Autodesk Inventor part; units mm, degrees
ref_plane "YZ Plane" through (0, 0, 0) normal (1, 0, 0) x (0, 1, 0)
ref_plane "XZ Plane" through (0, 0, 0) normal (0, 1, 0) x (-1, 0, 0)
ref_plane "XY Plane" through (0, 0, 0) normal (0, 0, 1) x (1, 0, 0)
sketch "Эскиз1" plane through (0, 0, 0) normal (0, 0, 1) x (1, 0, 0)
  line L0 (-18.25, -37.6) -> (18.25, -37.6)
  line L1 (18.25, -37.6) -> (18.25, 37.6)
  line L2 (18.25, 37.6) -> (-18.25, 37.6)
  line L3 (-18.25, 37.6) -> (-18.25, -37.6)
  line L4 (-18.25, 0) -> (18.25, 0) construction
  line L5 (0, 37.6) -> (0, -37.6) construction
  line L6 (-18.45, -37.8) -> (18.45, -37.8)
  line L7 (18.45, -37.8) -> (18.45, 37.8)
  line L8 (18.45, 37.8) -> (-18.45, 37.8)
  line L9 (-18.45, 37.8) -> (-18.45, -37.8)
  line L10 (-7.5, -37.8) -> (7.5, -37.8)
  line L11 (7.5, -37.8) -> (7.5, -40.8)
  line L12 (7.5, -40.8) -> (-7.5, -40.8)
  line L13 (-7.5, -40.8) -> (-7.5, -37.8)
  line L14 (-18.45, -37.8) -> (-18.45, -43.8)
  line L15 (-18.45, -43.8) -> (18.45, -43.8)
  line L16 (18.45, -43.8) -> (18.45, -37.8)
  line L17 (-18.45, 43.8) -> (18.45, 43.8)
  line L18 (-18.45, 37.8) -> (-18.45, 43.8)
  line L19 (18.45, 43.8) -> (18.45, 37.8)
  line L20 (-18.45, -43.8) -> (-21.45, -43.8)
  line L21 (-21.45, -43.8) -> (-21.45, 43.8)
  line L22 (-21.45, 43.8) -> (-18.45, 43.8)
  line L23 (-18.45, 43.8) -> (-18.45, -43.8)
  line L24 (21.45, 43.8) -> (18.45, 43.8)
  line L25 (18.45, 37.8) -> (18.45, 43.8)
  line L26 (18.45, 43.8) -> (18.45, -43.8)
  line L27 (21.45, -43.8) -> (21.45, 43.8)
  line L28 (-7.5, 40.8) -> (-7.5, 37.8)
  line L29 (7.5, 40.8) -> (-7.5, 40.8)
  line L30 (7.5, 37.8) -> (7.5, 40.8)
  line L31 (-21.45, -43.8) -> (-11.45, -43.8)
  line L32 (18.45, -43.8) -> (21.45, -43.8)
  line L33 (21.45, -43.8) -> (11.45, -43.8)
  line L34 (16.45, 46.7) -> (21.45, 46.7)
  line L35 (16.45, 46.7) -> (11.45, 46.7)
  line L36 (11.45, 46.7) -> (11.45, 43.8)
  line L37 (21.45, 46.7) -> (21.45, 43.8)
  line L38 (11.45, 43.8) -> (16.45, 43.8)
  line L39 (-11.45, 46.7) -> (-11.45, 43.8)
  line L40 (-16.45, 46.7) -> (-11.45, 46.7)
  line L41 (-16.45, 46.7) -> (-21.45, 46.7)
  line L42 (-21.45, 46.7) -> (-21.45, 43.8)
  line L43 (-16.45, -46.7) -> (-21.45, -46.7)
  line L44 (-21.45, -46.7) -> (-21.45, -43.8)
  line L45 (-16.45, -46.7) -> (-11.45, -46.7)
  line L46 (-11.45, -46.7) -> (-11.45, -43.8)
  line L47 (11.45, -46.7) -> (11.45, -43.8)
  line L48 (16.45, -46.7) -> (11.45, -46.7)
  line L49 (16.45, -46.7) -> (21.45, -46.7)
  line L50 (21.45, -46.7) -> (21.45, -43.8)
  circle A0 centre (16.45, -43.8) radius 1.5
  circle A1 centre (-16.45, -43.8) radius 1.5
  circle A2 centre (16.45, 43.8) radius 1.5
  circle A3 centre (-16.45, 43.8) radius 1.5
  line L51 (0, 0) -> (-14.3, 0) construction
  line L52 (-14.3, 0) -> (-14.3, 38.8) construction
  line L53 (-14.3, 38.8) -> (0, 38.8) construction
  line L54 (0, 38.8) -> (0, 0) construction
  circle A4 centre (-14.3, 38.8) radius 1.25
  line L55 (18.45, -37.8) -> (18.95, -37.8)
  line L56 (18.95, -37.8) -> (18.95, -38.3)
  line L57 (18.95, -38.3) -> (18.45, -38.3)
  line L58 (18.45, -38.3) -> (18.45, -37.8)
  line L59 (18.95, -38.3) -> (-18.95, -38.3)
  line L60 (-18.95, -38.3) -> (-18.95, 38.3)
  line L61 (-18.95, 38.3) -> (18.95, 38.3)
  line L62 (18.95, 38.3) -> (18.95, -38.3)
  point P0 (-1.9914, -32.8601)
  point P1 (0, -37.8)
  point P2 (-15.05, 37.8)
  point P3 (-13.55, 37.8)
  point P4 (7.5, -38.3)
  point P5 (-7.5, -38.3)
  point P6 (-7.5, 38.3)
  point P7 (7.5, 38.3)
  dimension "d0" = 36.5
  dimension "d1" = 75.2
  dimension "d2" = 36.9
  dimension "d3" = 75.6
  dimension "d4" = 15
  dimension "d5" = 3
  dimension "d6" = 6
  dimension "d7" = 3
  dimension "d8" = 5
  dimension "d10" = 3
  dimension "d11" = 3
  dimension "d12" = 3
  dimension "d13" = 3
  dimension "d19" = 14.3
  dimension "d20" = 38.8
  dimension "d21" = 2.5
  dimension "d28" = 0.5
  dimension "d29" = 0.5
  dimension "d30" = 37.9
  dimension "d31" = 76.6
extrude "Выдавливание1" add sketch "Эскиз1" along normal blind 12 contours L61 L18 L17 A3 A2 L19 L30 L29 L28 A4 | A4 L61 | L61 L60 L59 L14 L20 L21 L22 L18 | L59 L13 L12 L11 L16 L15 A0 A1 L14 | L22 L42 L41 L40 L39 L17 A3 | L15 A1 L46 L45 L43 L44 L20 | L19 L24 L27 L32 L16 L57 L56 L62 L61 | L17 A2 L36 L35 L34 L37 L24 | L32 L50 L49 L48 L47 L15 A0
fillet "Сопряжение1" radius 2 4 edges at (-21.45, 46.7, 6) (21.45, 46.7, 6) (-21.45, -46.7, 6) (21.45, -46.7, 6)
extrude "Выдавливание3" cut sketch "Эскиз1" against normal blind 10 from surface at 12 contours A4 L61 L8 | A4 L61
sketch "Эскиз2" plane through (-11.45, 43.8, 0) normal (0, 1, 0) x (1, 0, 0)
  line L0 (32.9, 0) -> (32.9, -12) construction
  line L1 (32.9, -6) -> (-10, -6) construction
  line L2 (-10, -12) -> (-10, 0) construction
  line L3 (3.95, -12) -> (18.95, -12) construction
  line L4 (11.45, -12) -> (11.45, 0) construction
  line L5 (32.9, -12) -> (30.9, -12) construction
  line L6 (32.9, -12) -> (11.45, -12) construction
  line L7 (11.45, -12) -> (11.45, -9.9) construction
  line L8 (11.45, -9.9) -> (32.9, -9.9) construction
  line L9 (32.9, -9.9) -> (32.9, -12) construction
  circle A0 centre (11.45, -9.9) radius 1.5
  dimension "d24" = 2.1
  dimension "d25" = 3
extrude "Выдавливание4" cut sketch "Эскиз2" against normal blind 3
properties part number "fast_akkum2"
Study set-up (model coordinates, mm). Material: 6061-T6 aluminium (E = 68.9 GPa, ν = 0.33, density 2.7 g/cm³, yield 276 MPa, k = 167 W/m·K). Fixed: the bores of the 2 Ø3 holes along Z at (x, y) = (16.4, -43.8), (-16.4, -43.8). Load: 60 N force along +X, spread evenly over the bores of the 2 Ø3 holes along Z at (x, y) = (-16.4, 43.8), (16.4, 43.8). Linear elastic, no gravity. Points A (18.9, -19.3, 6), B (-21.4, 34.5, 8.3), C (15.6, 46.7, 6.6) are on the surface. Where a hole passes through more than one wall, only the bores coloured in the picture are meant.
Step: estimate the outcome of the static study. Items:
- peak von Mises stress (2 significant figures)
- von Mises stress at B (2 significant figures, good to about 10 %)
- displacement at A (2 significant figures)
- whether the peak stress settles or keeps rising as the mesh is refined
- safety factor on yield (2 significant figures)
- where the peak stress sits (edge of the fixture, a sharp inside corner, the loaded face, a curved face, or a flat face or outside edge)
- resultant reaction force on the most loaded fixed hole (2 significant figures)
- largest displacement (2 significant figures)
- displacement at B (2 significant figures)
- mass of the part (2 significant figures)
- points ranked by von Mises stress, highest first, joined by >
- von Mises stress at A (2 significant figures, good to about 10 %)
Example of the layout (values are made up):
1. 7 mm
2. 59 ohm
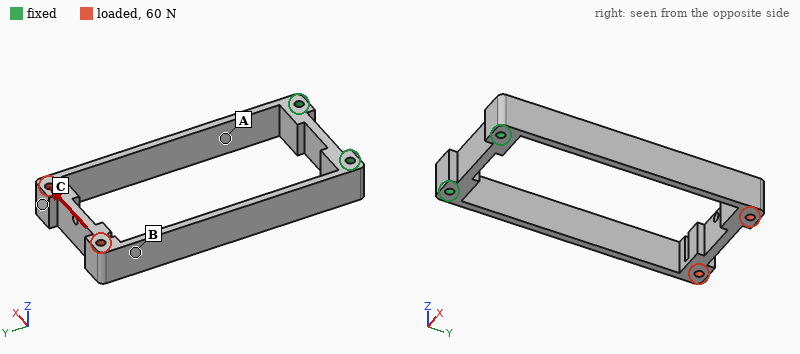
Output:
1. 92 MPa
2. 74 MPa
3. 0.19 mm
4. settles
5. 3.0
6. a flat face or outside edge
7. 82 N
8. 1.2 mm
9. 1.2 mm
10. 28 g
11. B > A > C
12. 45 MPa
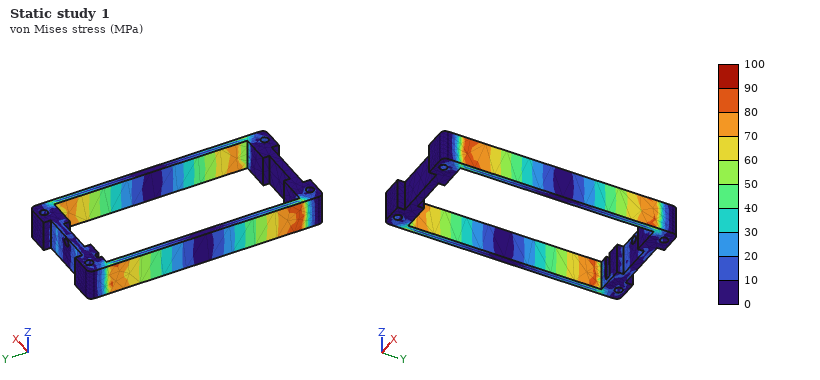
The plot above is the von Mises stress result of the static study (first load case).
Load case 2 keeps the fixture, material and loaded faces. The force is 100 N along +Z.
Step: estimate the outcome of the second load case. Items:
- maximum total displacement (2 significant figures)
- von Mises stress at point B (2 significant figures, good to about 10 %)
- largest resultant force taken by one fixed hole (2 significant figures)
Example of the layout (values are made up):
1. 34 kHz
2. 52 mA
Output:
1. 0.47 mm
2. 5.5 MPa
3. 50 N
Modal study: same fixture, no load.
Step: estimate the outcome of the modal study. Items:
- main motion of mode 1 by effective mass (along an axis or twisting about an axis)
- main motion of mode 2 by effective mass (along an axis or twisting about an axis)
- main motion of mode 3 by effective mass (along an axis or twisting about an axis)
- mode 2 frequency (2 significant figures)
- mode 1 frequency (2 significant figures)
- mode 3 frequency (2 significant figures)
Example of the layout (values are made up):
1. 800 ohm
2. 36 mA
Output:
1. along X
2. along Z
3. twisting about Y
4. 760 Hz
5. 320 Hz
6. 1300 Hz
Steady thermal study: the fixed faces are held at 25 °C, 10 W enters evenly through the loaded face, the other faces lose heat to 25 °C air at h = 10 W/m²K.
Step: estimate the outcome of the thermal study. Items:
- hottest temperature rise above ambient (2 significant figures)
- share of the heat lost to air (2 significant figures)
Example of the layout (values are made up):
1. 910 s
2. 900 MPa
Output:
1. 66 K
2. 26 %
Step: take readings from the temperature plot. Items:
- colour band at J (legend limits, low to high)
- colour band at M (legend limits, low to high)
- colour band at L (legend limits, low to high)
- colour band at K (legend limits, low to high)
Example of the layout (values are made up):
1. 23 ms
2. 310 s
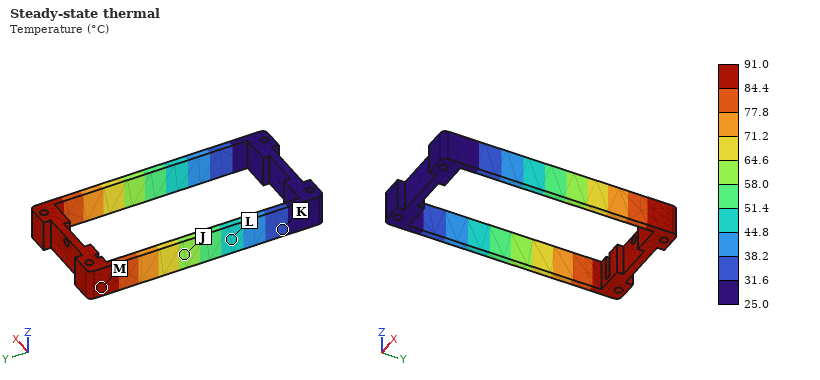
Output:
1. 58.0 to 64.6 °C
2. 84.4 to 91.0 °C
3. 44.8 to 51.4 °C
4. 31.6 to 38.2 °C
